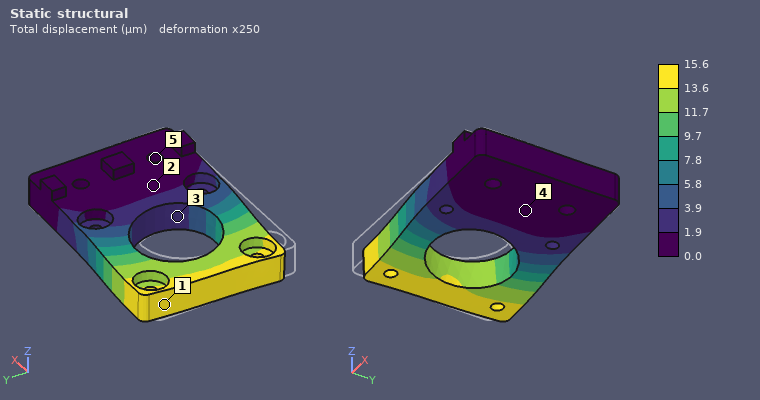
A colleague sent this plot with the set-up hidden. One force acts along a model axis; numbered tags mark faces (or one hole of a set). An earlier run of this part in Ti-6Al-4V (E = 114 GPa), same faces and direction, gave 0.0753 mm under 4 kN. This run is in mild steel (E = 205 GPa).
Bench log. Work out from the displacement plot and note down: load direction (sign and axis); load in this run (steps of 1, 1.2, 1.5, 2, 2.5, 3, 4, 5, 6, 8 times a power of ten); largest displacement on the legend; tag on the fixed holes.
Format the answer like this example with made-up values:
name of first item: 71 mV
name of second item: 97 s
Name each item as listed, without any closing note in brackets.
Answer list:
load direction: +Y
load in this run: 1.5 kN
largest displacement on the legend: 15.6 µm
tag on the fixed holes: 5
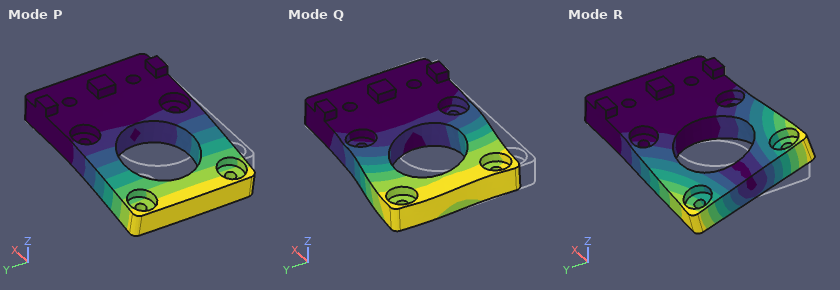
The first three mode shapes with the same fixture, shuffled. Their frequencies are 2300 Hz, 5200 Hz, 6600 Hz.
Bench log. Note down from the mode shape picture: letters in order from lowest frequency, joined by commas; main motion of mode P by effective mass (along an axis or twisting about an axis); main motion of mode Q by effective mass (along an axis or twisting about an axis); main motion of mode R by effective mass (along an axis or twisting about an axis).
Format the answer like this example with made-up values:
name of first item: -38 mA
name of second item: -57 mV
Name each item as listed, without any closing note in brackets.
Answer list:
letters in order from lowest frequency, joined by commas: P, R, Q
main motion of mode P by effective mass: along Z
main motion of mode Q by effective mass: along Y
main motion of mode R by effective mass: twisting about X
